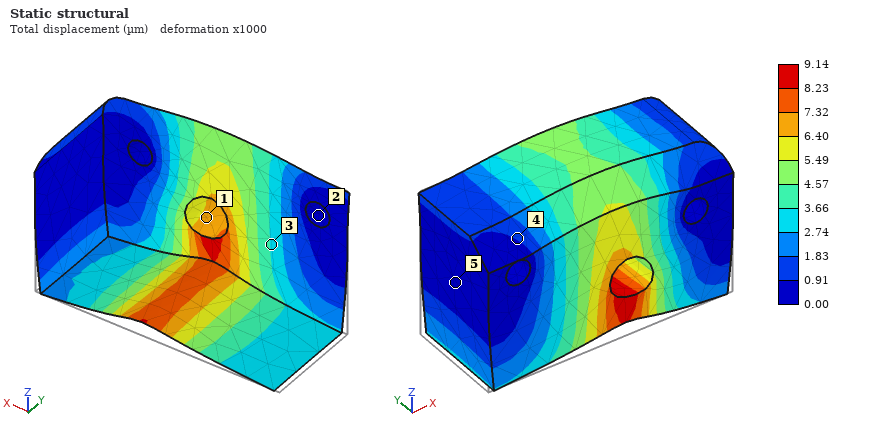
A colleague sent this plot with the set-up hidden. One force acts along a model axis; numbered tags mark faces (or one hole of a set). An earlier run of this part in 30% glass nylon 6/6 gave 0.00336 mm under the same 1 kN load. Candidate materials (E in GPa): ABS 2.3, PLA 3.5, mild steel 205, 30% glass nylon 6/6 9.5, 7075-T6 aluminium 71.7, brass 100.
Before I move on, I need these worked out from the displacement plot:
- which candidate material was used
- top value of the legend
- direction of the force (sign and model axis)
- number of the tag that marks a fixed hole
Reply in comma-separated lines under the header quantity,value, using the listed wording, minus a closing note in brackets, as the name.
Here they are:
quantity,value
which candidate material was used,PLA
top value of the legend,9.14 µm
direction of the force,+Z
number of the tag that marks a fixed hole,2
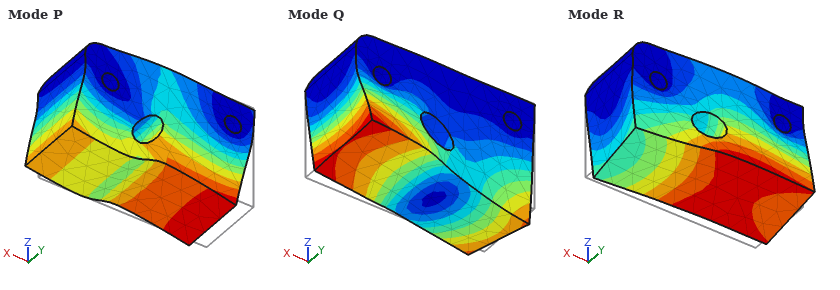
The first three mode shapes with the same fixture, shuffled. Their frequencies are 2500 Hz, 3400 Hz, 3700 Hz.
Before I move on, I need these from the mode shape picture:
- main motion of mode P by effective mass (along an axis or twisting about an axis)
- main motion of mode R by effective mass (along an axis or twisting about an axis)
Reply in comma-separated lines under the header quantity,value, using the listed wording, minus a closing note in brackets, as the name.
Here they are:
quantity,value
main motion of mode P by effective mass,along X
main motion of mode R by effective mass,along Y
